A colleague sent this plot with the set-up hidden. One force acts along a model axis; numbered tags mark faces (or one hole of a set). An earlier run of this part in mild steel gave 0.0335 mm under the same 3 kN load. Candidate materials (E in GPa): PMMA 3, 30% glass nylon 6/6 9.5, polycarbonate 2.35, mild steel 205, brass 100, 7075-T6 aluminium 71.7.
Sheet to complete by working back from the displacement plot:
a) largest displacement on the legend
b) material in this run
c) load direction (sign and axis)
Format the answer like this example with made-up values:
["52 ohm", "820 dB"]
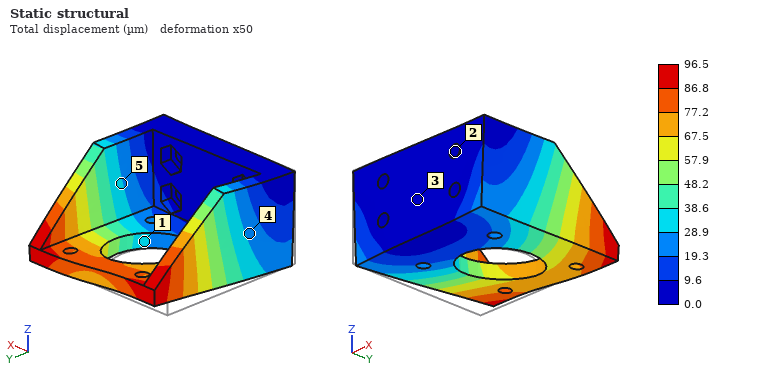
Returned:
["96.5 µm", "7075-T6 aluminium", "+X"]
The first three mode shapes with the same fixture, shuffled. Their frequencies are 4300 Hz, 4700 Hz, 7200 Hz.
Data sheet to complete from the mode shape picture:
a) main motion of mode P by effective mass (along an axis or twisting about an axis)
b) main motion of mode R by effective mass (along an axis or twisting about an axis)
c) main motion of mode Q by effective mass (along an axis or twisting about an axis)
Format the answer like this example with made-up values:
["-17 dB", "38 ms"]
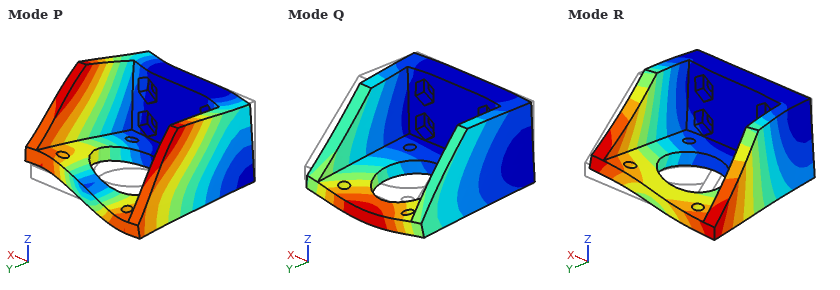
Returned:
["along X", "along X", "along Z"]
